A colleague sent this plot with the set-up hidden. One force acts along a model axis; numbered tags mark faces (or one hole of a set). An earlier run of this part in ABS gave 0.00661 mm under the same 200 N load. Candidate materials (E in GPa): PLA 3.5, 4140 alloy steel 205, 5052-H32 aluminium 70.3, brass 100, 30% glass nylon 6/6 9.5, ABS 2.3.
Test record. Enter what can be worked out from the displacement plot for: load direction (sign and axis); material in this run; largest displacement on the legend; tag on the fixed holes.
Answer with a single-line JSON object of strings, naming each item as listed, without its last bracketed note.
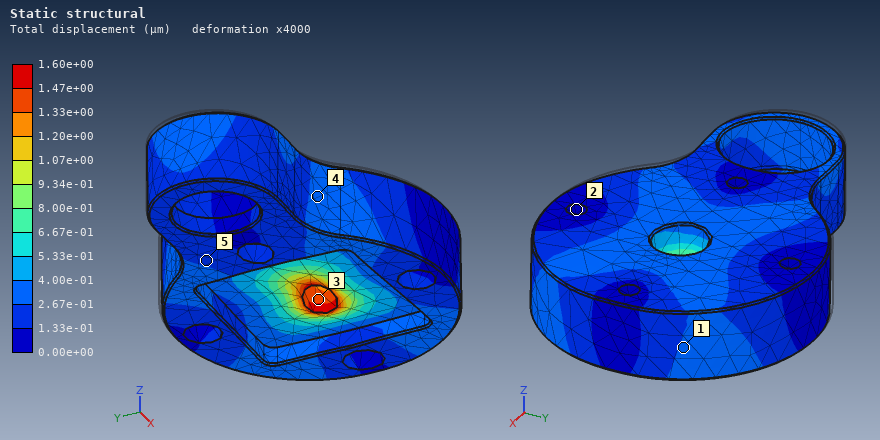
{"load direction": "+X", "material in this run": "30% glass nylon 6/6", "largest displacement on the legend": "1.60e+00 µm", "tag on the fixed holes": "2"}
